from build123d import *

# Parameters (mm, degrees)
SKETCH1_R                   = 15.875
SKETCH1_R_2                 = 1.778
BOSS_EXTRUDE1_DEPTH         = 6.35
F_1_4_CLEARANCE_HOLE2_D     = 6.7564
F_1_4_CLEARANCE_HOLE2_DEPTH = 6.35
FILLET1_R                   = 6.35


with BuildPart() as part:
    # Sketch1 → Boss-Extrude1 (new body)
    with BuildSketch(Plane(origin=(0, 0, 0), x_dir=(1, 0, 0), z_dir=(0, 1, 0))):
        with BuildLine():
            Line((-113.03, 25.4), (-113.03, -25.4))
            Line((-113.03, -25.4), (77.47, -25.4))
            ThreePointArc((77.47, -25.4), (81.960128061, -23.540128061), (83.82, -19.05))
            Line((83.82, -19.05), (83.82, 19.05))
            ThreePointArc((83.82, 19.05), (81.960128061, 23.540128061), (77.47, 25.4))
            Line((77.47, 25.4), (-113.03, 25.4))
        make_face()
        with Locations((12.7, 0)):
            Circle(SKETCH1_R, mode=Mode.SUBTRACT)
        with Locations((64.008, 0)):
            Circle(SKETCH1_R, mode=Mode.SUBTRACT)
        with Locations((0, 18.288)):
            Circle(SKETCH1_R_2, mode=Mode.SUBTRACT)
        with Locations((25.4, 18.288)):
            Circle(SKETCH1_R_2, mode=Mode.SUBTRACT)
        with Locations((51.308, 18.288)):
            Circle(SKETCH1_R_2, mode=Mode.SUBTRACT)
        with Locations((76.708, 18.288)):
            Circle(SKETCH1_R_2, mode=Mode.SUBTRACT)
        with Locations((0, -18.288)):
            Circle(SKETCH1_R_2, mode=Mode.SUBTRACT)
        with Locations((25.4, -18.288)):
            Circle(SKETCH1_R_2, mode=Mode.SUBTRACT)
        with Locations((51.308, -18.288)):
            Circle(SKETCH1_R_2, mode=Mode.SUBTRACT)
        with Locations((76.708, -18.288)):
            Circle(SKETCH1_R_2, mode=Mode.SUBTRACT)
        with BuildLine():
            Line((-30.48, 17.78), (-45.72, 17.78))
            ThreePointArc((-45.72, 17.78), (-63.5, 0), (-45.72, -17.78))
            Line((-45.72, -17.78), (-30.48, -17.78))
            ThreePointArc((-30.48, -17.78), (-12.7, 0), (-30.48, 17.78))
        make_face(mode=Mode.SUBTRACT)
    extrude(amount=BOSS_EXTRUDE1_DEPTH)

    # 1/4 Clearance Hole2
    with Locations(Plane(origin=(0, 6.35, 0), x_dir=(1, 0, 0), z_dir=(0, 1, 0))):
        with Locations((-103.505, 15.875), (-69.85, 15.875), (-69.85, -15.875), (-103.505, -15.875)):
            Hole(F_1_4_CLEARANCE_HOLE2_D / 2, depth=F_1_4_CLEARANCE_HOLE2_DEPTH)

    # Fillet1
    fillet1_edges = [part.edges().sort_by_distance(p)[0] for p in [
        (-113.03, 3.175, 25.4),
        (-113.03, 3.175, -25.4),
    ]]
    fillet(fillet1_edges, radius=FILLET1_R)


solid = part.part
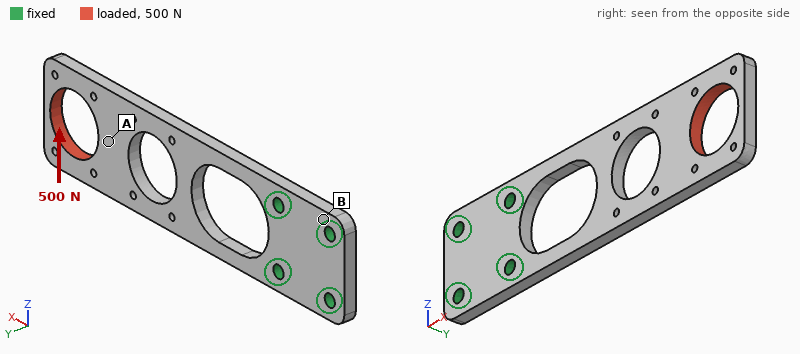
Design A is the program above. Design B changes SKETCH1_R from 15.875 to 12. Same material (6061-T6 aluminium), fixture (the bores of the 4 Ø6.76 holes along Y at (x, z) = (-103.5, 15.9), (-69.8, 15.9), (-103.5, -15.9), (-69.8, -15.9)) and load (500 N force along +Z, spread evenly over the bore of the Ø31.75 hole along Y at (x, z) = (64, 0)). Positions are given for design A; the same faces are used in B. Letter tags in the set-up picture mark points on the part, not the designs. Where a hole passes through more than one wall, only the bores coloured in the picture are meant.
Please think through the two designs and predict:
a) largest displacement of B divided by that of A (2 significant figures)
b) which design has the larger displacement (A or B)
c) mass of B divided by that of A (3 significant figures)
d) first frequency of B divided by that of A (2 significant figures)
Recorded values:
0.90
A
1.10
0.91
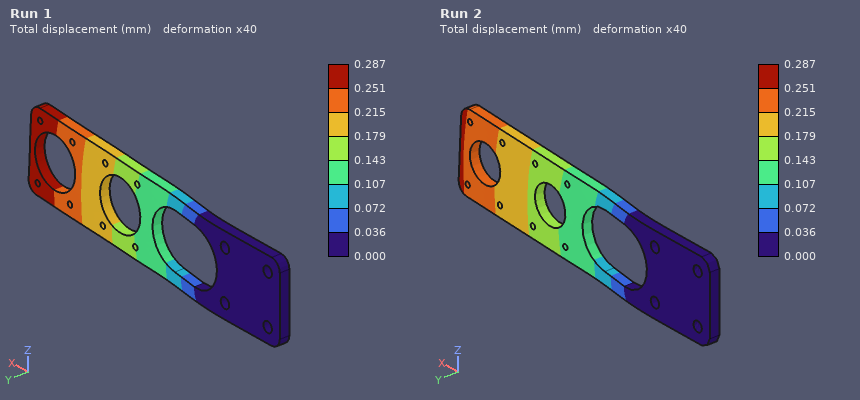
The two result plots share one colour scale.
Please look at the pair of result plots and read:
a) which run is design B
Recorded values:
Run 2
